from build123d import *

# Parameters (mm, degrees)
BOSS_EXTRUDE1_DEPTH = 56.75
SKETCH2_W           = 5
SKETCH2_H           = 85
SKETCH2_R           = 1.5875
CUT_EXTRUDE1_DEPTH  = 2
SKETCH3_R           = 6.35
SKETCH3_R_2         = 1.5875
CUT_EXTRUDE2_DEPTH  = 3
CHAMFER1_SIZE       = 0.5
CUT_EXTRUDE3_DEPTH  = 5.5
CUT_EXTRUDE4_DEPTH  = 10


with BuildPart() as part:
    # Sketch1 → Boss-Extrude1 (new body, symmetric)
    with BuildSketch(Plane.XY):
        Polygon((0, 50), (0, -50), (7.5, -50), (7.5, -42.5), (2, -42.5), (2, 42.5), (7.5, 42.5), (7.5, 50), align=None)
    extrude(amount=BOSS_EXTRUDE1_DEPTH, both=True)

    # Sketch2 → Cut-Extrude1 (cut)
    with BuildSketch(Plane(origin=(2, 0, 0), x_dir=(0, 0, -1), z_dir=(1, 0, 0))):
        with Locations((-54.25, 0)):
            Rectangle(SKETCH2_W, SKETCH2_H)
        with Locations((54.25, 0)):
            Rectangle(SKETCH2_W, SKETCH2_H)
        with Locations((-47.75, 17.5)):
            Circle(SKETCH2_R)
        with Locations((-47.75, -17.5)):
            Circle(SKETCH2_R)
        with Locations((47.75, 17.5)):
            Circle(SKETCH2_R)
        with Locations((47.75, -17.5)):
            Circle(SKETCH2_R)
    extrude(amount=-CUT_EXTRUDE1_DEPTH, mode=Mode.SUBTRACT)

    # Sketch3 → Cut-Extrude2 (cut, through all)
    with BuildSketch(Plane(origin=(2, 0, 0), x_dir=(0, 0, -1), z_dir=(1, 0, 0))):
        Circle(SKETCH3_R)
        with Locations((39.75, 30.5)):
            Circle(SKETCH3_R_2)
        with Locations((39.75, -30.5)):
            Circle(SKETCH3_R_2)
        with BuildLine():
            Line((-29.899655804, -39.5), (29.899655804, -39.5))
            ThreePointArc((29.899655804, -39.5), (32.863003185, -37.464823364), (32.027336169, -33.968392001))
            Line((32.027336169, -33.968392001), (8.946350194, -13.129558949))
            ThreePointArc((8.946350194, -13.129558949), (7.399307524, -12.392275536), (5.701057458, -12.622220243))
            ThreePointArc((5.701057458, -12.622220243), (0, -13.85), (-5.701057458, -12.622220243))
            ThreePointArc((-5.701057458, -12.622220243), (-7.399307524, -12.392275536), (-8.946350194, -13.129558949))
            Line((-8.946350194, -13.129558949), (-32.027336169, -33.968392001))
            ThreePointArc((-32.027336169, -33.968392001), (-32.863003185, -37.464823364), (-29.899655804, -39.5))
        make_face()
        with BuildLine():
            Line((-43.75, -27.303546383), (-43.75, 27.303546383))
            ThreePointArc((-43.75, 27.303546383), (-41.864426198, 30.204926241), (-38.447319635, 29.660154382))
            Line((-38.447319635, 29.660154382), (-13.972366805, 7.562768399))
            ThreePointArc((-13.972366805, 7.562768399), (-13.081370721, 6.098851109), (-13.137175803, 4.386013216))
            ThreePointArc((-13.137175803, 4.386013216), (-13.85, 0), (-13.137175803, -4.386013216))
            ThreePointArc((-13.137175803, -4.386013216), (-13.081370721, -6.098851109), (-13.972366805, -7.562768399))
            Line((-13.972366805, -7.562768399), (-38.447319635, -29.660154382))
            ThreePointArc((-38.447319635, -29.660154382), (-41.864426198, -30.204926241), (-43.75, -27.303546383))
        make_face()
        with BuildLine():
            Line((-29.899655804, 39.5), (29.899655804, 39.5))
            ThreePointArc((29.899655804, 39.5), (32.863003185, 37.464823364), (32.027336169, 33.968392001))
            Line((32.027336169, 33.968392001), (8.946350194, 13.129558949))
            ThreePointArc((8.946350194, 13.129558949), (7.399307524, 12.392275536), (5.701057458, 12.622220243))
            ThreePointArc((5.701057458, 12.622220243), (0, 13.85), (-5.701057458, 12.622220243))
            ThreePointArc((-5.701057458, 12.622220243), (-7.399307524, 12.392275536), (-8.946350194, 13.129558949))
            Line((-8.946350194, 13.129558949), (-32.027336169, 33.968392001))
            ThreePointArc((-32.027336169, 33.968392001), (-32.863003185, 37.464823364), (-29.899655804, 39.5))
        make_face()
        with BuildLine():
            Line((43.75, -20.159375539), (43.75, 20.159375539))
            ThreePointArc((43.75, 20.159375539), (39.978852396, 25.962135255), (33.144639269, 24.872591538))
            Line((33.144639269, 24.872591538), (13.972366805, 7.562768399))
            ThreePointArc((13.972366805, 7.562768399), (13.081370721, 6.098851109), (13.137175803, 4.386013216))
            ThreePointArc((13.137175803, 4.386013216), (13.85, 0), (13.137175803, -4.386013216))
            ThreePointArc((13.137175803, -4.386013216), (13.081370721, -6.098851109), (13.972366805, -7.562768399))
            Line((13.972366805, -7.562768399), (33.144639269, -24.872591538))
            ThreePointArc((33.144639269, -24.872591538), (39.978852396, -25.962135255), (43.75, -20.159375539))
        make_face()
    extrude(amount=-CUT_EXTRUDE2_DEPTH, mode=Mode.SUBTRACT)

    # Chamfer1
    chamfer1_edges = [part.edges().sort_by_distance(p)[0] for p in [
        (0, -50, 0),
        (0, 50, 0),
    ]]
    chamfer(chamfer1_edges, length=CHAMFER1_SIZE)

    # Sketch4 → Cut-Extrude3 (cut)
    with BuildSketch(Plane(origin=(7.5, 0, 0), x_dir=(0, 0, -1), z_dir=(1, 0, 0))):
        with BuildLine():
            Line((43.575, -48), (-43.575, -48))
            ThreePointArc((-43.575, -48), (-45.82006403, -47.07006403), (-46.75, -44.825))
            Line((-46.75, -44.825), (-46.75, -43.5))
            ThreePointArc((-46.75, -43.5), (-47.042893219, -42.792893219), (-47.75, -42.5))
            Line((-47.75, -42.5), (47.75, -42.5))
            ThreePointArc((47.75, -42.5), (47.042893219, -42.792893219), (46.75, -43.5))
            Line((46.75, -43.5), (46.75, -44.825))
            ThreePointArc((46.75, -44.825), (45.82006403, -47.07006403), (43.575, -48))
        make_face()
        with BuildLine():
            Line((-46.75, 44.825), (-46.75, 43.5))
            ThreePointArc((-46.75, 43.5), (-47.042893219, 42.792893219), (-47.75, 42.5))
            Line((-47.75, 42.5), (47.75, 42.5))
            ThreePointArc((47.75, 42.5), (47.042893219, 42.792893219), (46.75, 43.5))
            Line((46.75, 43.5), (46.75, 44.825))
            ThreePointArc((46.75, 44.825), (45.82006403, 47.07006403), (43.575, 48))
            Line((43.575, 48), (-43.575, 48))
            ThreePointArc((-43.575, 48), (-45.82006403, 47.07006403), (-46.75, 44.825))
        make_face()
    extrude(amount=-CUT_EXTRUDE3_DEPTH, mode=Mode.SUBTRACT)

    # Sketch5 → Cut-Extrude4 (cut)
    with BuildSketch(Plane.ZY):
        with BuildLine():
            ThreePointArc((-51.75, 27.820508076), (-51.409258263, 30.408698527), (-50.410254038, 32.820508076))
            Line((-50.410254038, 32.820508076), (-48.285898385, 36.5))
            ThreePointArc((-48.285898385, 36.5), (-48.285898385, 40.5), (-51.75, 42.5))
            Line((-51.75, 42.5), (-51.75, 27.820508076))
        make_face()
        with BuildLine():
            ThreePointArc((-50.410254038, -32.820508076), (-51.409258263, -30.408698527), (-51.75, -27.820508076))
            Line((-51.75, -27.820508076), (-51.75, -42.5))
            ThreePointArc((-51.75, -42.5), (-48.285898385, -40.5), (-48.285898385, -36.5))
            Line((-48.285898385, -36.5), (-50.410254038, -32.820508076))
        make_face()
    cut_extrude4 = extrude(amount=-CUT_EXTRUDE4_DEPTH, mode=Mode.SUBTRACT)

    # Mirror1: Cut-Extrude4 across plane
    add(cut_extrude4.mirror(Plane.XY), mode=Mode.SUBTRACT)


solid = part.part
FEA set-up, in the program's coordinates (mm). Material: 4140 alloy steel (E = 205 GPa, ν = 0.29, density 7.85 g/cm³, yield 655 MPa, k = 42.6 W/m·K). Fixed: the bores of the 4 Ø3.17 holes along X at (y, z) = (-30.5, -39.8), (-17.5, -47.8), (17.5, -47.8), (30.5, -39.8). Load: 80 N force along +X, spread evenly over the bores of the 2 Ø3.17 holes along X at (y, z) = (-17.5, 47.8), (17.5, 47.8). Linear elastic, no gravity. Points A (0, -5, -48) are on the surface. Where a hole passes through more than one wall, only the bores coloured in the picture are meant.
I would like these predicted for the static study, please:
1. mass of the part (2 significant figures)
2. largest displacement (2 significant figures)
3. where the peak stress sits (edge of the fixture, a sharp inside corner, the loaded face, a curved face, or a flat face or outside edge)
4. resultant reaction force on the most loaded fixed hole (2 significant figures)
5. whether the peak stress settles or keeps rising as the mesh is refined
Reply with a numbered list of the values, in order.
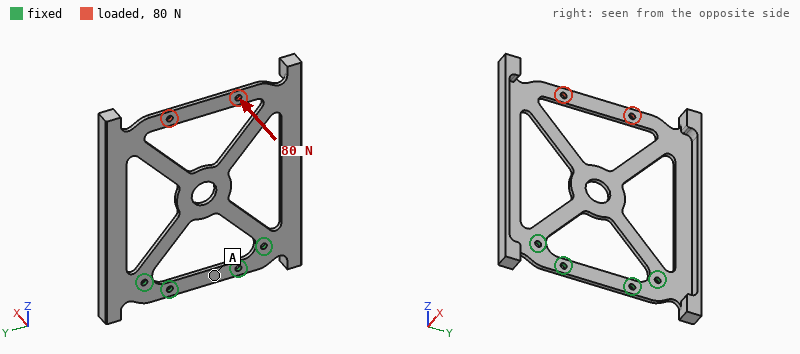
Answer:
1. 110 g
2. 1.6 mm
3. edge of the fixture
4. 130 N
5. keeps rising
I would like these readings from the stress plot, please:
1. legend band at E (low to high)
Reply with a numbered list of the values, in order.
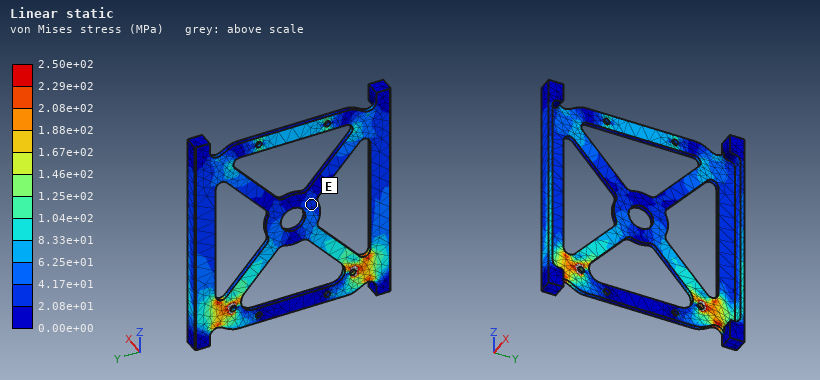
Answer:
1. 2.08e+01 to 4.17e+01 MPa
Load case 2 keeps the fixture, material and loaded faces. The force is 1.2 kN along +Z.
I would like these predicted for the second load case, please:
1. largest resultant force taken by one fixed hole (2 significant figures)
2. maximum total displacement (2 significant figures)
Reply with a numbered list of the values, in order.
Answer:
1. 940 N
2. 0.14 mm
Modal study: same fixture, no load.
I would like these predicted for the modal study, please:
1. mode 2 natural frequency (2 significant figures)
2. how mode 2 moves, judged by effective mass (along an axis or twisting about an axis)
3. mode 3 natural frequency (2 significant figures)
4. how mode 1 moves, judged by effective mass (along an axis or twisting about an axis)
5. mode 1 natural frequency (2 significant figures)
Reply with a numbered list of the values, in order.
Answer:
1. 290 Hz
2. twisting about Z
3. 770 Hz
4. along X
5. 200 Hz
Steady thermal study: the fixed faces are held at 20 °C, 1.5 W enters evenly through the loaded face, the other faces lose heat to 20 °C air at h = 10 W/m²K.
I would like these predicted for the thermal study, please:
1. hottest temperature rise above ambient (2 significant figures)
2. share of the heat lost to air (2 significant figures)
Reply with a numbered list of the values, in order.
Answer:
1. 32 K
2. 76 %
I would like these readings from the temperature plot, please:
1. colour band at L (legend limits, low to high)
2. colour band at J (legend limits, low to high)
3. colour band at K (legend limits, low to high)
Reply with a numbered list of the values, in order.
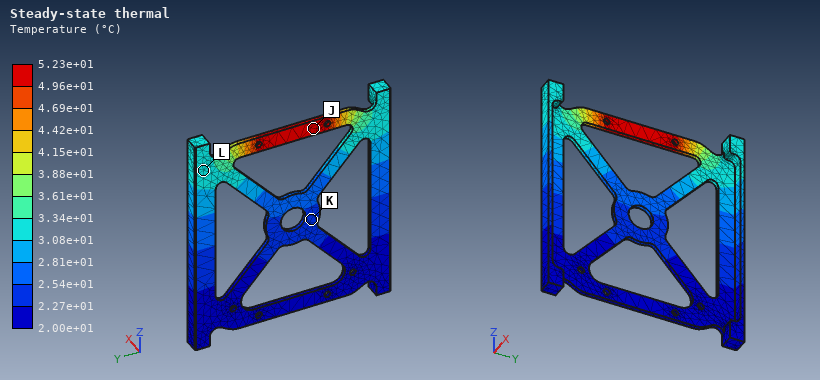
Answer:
1. 3.08e+01 to 3.34e+01 °C
2. 4.96e+01 to 5.23e+01 °C
3. 2.27e+01 to 2.54e+01 °C
